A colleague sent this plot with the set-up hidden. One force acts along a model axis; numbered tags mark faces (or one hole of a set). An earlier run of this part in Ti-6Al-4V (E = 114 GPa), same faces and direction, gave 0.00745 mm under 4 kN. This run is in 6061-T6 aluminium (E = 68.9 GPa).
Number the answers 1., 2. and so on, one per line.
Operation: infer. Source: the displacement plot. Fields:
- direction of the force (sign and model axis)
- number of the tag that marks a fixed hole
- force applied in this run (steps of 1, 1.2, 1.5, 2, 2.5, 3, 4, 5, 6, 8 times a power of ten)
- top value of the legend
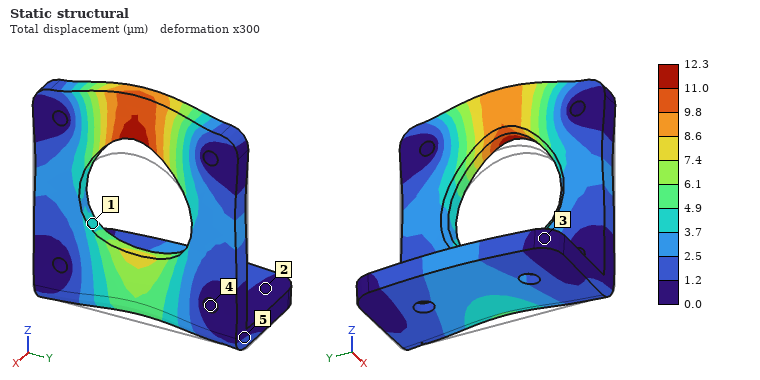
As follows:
1. +Z
2. 4
3. 4 kN
4. 12.3 µm
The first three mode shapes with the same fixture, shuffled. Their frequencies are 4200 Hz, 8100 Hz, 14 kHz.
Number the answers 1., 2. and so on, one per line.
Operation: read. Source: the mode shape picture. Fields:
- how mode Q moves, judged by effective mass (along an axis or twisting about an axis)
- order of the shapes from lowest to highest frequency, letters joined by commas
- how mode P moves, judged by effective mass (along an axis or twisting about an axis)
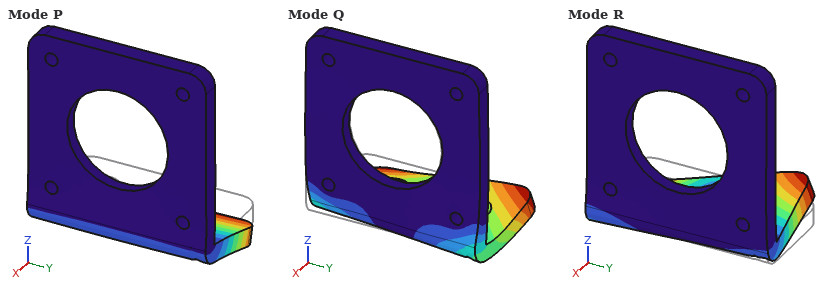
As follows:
1. along Y
2. P, R, Q
3. along Z
